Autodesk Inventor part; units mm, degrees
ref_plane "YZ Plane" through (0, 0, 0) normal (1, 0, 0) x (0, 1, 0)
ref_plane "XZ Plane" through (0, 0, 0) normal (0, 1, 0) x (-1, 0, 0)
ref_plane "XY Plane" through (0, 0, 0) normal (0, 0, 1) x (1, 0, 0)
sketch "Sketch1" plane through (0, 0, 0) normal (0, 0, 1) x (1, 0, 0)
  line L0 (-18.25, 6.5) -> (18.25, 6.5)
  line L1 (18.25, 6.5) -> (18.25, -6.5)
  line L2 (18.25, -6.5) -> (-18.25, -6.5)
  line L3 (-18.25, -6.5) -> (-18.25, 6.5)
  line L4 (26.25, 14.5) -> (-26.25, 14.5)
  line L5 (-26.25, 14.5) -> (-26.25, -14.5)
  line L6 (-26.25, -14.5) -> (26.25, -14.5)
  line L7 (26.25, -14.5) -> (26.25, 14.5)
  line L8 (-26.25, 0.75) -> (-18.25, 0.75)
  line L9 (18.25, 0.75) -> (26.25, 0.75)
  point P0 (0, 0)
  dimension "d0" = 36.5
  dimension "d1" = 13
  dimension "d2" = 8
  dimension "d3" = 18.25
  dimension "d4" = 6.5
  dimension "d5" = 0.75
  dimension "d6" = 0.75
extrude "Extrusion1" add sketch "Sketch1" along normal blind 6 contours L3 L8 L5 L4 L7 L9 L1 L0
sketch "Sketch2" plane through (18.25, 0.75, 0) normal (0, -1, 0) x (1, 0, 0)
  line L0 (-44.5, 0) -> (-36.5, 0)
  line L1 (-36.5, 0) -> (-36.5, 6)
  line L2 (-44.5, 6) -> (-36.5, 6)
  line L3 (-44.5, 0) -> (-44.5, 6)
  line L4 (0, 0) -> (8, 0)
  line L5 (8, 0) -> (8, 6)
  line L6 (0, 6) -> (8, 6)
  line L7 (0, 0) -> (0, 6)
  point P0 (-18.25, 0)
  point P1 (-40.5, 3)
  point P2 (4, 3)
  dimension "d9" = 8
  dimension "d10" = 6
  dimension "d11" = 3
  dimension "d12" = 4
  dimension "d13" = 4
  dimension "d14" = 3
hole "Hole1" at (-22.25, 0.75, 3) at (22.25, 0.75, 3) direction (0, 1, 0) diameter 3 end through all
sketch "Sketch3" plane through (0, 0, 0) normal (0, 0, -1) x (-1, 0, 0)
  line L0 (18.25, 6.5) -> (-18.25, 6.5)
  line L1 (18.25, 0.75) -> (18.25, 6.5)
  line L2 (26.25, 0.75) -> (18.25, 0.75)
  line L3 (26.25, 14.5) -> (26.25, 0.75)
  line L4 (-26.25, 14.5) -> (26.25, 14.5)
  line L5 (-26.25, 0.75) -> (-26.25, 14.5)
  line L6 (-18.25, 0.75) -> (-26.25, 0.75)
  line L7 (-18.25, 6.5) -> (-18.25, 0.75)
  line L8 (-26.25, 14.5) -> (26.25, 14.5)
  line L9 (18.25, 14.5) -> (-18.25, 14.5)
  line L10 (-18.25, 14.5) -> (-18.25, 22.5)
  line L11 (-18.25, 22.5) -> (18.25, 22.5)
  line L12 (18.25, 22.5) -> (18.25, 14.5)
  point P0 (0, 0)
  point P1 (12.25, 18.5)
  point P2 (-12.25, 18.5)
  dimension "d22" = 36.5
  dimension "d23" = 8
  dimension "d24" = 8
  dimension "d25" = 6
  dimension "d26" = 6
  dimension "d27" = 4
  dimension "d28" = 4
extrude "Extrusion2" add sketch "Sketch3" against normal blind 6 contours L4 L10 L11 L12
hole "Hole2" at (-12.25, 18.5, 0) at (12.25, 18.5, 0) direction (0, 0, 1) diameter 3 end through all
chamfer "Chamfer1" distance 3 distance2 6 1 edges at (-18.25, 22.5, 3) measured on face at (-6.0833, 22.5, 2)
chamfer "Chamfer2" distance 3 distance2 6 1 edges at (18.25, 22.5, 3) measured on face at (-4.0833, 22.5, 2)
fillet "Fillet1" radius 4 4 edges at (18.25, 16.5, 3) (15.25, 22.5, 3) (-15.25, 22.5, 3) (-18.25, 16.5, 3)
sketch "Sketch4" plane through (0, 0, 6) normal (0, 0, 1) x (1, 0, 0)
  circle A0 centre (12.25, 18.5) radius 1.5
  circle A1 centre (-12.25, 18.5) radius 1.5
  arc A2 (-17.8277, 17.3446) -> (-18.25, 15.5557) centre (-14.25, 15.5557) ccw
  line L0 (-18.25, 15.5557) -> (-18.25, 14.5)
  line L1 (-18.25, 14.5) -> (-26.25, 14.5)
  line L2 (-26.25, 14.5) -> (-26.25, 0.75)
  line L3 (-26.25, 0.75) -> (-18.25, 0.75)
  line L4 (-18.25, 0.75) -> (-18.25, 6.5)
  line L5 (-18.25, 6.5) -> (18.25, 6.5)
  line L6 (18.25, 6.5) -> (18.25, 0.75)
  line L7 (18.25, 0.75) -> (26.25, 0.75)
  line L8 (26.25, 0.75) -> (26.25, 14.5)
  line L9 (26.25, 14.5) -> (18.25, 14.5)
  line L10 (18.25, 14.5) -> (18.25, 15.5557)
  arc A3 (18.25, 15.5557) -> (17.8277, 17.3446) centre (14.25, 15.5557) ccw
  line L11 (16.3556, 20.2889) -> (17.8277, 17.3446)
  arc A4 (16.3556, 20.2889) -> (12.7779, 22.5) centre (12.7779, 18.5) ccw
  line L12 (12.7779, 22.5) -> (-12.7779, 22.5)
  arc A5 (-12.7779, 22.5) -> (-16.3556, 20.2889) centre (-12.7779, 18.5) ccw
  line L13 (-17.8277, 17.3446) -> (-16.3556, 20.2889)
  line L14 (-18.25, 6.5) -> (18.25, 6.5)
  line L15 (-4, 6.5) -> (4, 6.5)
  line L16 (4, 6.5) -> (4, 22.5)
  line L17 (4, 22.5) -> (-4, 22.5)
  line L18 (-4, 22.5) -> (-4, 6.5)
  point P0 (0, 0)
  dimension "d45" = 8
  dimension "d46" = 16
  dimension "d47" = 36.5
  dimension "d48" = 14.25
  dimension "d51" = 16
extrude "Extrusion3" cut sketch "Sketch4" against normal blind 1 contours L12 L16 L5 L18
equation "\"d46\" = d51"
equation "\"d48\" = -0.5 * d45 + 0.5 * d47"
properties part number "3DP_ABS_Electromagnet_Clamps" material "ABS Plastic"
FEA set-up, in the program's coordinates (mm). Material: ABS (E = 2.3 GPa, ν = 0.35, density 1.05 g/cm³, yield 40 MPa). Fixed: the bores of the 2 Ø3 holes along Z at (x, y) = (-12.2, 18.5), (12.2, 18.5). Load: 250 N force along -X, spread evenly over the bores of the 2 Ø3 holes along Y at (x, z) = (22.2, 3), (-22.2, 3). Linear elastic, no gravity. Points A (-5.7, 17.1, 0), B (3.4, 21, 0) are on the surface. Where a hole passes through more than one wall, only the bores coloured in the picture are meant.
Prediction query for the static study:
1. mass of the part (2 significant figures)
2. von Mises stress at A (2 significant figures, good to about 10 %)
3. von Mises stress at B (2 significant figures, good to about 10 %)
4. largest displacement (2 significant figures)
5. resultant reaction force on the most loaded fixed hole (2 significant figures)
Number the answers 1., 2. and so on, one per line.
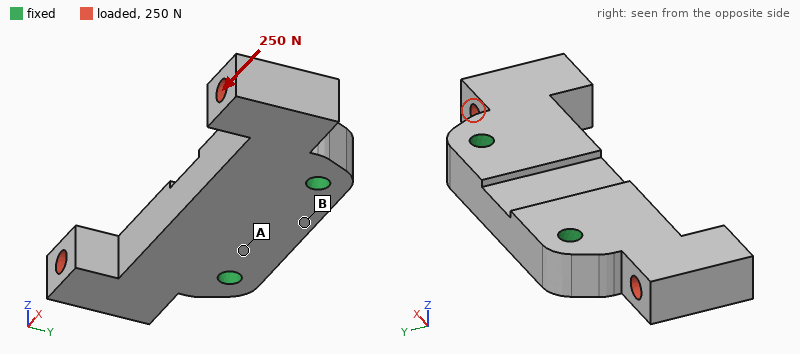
1. 4.5 g
2. 2.5 MPa
3. 1.1 MPa
4. 0.14 mm
5. 160 N
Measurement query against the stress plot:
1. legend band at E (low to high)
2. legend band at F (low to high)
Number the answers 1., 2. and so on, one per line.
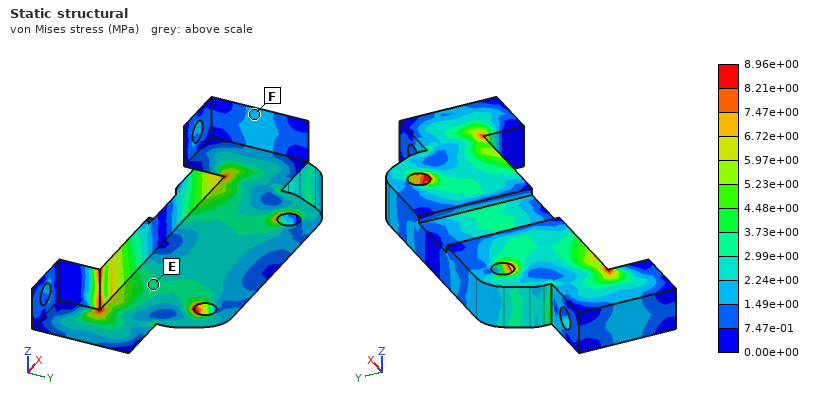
1. 2.99e+00 to 3.73e+00 MPa
2. 1.49e+00 to 2.24e+00 MPa
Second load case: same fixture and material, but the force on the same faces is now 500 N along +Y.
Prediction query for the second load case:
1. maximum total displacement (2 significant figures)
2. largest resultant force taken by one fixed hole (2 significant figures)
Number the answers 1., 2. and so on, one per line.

1. 0.32 mm
2. 320 N
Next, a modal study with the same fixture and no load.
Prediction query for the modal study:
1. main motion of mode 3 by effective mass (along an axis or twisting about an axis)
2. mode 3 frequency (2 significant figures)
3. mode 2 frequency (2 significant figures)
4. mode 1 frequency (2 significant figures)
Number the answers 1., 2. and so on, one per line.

1. along X
2. 5600 Hz
3. 3600 Hz
4. 3500 Hz
